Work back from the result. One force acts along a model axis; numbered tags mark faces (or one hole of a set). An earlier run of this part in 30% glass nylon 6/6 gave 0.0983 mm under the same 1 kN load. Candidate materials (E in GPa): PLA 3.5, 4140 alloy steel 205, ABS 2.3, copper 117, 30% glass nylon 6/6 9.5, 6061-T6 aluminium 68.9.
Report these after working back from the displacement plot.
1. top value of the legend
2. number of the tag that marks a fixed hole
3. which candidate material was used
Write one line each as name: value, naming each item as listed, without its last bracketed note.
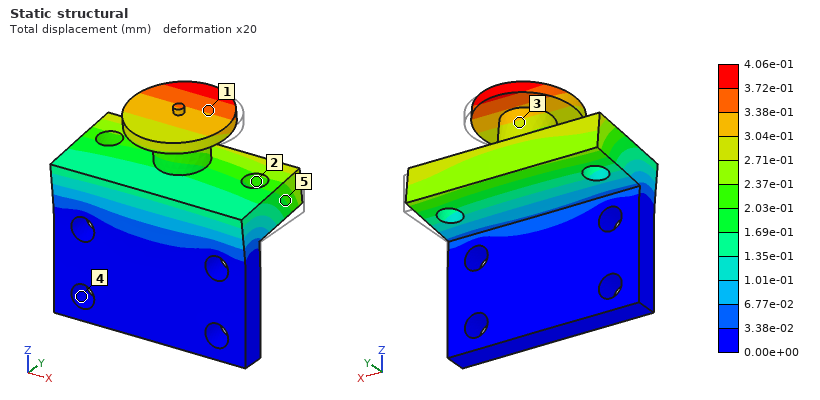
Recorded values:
top value of the legend: 4.06e-01 mm
number of the tag that marks a fixed hole: 4
which candidate material was used: ABS
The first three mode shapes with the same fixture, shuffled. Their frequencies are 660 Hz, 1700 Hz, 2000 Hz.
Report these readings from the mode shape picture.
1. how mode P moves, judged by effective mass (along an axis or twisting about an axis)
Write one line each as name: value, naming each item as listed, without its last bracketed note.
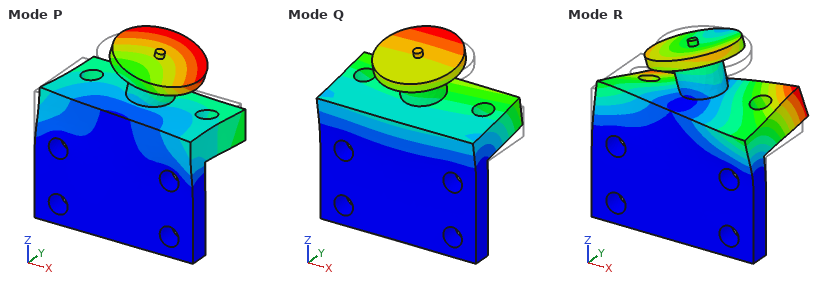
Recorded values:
how mode P moves, judged by effective mass: along X
